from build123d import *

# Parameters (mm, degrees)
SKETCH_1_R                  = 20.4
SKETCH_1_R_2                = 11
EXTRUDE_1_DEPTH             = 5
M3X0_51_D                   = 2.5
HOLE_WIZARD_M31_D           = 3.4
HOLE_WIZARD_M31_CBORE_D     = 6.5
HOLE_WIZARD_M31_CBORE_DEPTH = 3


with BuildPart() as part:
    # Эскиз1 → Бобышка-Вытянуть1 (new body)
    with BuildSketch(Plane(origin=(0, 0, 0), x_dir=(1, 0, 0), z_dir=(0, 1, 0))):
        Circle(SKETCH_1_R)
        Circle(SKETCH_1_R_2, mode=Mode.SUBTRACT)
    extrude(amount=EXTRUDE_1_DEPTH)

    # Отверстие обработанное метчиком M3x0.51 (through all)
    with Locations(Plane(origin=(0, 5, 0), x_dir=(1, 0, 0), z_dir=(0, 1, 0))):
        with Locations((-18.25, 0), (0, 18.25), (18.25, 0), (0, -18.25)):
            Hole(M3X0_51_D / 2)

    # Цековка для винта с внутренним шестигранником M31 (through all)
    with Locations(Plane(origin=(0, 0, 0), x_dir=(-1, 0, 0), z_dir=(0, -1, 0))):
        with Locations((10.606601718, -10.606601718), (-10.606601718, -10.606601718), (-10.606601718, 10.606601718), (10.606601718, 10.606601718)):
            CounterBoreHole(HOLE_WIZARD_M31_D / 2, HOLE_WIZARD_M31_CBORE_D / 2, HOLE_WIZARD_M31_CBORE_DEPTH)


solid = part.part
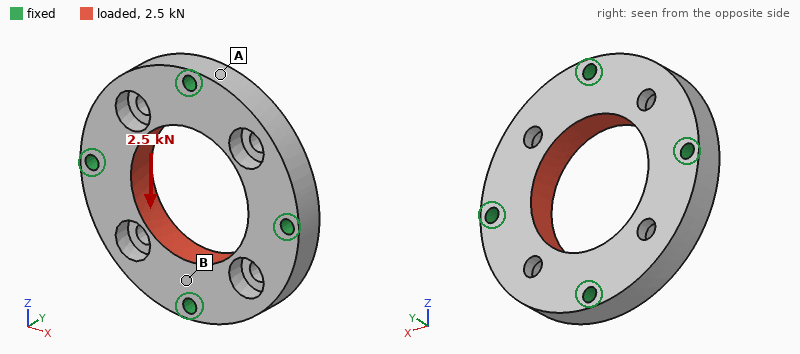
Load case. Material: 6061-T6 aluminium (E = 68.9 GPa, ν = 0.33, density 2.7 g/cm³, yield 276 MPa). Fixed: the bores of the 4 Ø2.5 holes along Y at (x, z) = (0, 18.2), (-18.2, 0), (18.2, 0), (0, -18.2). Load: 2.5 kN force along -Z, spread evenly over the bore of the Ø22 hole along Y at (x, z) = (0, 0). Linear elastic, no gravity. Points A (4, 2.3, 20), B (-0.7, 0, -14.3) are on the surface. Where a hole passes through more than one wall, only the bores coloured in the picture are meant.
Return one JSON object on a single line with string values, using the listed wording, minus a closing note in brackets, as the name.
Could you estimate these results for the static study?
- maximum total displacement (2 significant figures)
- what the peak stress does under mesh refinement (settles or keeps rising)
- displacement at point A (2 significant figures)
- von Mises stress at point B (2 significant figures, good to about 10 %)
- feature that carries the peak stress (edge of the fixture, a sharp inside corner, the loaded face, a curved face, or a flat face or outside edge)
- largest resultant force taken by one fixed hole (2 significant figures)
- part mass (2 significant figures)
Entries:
{"maximum total displacement": "6.3 µm", "what the peak stress does under mesh refinement": "keeps rising", "displacement at point A": "1.2 µm", "von Mises stress at point B": "15 MPa", "feature that carries the peak stress": "edge of the fixture", "largest resultant force taken by one fixed hole": "630 N", "part mass": "11 g"}
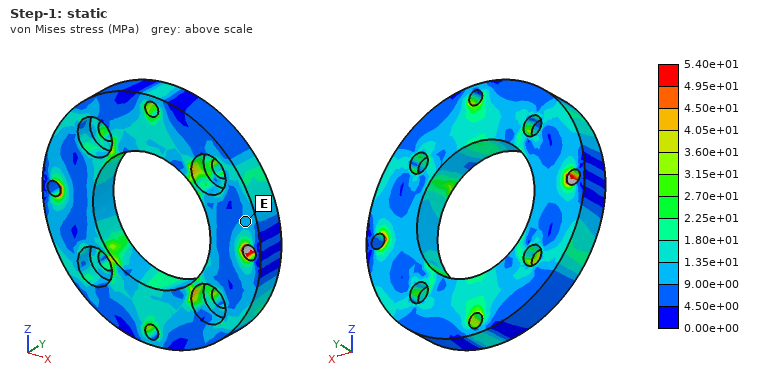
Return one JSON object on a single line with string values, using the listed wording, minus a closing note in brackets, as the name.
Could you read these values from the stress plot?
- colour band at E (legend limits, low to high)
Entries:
{"colour band at E": "9.00e+00 to 1.35e+01 MPa"}
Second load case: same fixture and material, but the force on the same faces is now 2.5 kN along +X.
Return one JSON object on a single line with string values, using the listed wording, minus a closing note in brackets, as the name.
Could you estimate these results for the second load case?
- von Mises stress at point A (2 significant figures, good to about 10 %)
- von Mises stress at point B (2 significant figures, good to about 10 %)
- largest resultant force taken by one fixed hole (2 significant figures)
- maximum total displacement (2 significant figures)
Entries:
{"von Mises stress at point A": "5.8 MPa", "von Mises stress at point B": "8.2 MPa", "largest resultant force taken by one fixed hole": "630 N", "maximum total displacement": "6.3 µm"}
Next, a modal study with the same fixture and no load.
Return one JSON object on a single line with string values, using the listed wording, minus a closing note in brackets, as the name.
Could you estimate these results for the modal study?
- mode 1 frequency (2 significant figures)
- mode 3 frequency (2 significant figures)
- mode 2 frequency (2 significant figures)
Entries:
{"mode 1 frequency": "27 kHz", "mode 3 frequency": "29 kHz", "mode 2 frequency": "29 kHz"}
